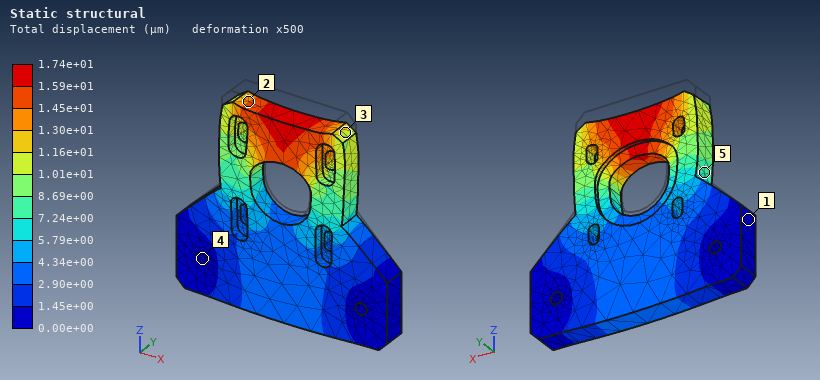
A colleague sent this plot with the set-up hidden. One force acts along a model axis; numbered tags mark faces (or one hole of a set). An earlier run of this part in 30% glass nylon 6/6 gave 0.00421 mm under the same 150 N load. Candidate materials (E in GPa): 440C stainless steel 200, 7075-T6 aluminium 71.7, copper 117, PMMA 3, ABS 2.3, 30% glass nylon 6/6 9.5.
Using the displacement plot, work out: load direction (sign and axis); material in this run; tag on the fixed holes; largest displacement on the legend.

-Z
ABS
4
1.74e+01 µm
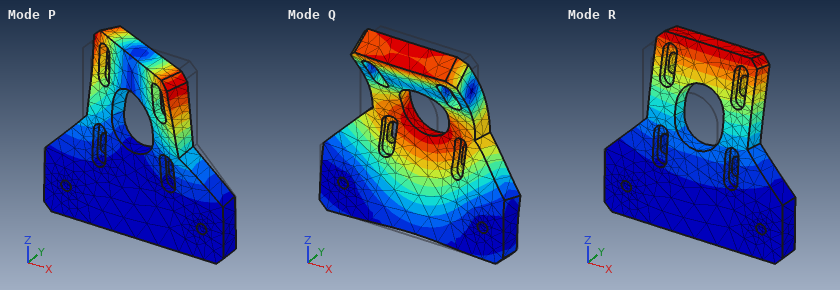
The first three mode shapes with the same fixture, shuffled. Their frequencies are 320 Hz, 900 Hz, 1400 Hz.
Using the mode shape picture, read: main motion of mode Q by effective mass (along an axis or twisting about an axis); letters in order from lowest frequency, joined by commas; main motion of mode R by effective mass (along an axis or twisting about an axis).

along Y
R, P, Q
along Y
